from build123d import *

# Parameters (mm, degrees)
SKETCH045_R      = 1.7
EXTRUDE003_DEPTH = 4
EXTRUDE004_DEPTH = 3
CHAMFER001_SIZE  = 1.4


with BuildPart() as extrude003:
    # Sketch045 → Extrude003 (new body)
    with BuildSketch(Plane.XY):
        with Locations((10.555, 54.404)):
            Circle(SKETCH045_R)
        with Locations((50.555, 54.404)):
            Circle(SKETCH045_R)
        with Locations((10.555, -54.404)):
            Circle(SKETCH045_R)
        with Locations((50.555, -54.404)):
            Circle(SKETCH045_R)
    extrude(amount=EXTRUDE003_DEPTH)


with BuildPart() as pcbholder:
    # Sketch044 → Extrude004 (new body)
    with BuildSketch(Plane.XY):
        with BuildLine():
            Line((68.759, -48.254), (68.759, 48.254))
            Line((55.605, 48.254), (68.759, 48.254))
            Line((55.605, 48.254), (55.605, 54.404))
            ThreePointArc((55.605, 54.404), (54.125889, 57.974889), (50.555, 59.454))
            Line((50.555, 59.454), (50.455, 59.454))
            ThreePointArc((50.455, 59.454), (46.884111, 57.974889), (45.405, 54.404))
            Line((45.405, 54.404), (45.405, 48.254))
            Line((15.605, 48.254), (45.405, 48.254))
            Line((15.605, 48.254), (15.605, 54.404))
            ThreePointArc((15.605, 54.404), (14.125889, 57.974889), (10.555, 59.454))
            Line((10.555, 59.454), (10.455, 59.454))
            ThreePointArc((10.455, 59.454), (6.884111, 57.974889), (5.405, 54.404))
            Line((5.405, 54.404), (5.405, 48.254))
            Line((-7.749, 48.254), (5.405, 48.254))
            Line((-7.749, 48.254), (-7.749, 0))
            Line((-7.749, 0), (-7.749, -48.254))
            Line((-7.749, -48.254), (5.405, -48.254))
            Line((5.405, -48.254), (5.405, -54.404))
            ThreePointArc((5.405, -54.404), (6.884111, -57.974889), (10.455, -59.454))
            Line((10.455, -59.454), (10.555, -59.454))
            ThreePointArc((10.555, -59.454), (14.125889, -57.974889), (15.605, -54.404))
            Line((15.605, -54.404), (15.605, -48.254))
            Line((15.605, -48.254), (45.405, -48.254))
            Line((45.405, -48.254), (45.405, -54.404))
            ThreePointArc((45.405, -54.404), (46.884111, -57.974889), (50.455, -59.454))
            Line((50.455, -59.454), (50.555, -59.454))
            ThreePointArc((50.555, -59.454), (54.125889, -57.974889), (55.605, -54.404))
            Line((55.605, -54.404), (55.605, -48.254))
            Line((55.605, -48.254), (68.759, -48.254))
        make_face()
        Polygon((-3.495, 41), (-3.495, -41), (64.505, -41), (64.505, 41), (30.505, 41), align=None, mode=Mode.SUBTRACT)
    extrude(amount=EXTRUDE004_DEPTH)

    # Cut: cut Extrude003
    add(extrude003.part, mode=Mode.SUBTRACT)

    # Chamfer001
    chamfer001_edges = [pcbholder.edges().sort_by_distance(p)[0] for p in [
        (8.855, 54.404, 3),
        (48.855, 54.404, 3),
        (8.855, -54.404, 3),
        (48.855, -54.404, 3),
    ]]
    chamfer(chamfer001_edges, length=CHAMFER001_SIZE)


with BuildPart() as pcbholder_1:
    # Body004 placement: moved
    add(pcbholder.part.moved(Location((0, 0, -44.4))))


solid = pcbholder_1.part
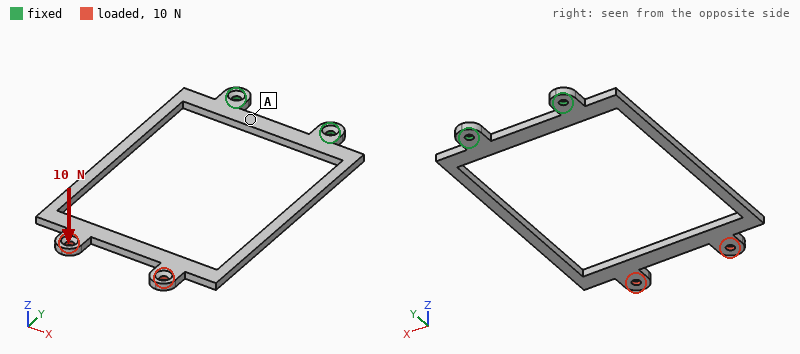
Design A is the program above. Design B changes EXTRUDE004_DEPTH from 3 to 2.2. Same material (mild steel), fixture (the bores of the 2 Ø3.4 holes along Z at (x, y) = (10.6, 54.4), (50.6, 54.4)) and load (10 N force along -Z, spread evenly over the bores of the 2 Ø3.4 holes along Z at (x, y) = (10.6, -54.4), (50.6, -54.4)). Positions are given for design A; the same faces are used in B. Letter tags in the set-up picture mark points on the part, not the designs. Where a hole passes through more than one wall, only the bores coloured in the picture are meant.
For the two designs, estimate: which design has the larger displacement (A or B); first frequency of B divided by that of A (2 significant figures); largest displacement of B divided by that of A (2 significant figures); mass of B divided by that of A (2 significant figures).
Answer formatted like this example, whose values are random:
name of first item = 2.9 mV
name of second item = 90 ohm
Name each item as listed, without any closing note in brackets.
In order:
which design has the larger displacement = B
first frequency of B divided by that of A = 0.74
largest displacement of B divided by that of A = 2.5
mass of B divided by that of A = 0.73
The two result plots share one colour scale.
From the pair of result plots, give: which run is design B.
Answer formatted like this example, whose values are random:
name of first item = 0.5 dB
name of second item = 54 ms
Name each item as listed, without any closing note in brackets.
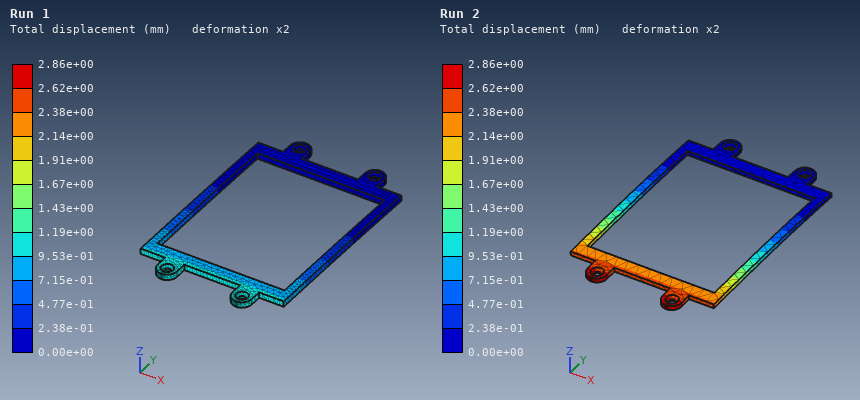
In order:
which run is design B = Run 2
